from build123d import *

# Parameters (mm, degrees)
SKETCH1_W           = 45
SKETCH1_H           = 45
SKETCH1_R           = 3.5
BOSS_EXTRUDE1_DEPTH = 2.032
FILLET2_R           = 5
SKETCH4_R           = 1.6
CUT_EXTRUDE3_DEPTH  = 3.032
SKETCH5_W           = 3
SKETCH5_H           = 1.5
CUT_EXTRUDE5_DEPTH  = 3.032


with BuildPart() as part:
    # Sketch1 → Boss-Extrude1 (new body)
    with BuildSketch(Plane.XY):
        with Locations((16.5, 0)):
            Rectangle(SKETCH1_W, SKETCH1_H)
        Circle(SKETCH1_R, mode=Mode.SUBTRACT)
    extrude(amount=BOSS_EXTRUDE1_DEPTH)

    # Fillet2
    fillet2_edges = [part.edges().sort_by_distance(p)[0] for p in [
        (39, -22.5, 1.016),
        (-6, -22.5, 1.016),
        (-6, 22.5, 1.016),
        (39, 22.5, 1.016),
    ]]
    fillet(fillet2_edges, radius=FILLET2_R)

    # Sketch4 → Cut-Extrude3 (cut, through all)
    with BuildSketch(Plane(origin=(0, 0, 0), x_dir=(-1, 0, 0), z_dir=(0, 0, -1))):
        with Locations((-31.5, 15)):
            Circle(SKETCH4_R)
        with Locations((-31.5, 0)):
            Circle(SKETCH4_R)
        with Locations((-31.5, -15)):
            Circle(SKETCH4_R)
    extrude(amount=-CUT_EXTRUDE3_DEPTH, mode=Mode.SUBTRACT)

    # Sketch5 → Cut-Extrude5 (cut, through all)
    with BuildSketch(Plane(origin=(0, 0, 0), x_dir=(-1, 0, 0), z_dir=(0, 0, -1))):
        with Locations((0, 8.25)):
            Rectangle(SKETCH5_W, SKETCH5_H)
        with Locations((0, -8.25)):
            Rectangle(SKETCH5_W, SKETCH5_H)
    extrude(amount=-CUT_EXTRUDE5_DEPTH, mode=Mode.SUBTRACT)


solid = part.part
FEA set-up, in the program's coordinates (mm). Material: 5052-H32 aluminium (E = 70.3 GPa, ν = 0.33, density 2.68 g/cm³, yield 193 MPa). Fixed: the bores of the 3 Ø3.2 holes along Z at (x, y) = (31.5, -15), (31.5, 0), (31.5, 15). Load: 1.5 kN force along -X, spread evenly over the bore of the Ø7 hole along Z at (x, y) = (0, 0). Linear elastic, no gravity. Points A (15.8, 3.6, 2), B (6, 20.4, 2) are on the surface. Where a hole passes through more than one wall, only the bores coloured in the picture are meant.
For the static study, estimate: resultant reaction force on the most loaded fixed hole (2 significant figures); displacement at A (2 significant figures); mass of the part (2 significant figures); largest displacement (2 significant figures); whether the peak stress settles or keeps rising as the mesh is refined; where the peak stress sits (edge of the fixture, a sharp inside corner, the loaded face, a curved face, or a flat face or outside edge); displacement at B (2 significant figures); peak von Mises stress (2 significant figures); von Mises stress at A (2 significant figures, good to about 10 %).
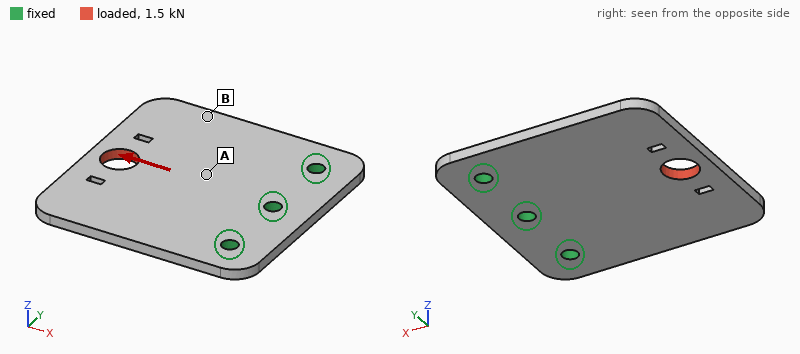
510 N
5.3 µm
11 g
22 µm
settles
the loaded face
4.0 µm
120 MPa
28 MPa
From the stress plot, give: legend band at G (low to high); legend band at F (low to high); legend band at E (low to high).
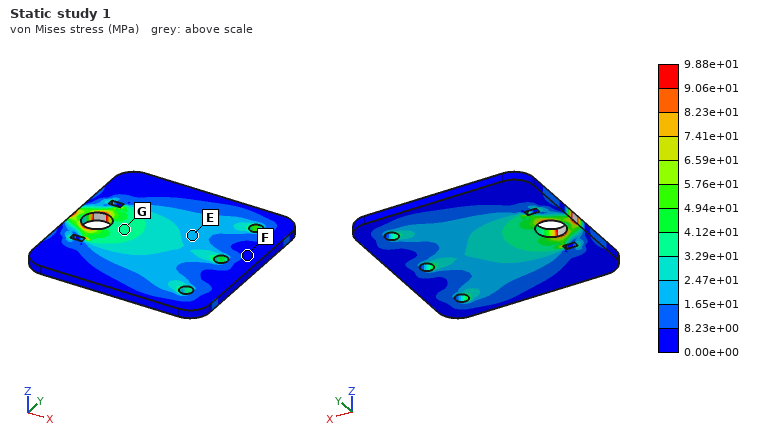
3.29e+01 to 4.12e+01 MPa
0.00e+00 to 8.23e+00 MPa
1.65e+01 to 2.47e+01 MPa
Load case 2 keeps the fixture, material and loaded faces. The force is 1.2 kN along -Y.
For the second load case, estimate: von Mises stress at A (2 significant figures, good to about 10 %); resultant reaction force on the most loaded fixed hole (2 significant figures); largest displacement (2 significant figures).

35 MPa
1.2 kN
43 µm
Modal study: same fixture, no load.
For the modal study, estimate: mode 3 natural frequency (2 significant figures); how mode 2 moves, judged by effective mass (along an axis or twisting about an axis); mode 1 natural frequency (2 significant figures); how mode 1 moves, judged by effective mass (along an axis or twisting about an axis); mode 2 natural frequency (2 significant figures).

6600 Hz
twisting about X
1300 Hz
along Z
2600 Hz
